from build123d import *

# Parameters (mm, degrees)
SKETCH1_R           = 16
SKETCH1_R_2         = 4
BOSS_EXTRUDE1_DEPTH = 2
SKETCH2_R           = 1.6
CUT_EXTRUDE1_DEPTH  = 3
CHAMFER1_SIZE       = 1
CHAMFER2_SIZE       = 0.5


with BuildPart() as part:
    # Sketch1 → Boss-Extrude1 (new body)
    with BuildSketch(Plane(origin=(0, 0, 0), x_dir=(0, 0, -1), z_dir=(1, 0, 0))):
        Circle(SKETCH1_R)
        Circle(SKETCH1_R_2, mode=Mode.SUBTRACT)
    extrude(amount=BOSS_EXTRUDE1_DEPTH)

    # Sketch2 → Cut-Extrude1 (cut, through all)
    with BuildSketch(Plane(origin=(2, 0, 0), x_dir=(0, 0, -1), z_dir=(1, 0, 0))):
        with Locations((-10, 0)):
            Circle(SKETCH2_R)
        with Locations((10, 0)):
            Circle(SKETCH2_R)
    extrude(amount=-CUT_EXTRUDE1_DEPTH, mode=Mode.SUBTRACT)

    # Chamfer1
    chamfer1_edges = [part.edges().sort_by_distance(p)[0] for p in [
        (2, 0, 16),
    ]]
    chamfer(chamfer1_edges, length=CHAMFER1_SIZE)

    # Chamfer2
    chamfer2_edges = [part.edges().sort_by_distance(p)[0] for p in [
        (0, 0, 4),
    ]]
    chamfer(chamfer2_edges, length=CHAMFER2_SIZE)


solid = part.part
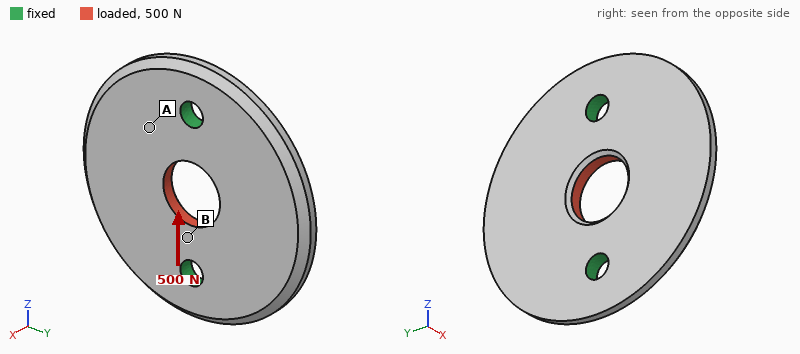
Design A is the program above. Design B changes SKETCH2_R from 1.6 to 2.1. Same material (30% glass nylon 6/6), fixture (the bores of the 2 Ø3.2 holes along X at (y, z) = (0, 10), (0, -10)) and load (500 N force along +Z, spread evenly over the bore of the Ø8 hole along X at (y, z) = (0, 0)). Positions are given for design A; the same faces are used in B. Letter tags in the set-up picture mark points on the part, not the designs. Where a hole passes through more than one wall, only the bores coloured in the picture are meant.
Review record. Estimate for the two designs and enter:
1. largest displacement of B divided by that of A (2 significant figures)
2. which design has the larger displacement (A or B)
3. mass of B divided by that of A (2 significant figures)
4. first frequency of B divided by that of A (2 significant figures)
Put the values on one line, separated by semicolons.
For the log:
0.91; A; 0.98; 1.1
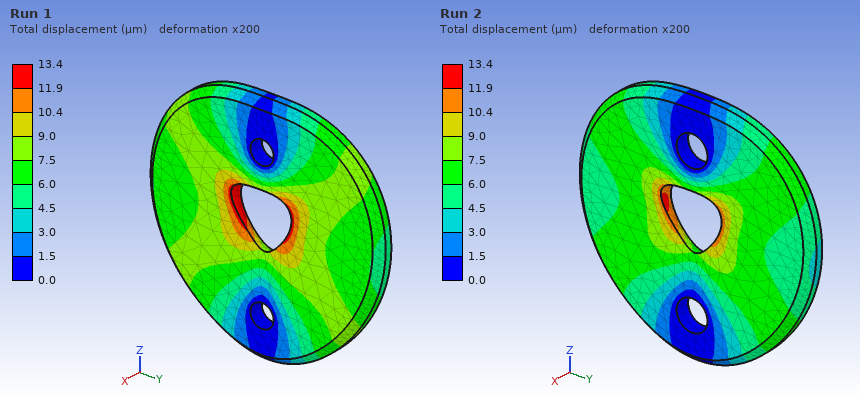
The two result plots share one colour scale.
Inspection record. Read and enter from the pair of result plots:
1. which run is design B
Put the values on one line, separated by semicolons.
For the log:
Run 2
